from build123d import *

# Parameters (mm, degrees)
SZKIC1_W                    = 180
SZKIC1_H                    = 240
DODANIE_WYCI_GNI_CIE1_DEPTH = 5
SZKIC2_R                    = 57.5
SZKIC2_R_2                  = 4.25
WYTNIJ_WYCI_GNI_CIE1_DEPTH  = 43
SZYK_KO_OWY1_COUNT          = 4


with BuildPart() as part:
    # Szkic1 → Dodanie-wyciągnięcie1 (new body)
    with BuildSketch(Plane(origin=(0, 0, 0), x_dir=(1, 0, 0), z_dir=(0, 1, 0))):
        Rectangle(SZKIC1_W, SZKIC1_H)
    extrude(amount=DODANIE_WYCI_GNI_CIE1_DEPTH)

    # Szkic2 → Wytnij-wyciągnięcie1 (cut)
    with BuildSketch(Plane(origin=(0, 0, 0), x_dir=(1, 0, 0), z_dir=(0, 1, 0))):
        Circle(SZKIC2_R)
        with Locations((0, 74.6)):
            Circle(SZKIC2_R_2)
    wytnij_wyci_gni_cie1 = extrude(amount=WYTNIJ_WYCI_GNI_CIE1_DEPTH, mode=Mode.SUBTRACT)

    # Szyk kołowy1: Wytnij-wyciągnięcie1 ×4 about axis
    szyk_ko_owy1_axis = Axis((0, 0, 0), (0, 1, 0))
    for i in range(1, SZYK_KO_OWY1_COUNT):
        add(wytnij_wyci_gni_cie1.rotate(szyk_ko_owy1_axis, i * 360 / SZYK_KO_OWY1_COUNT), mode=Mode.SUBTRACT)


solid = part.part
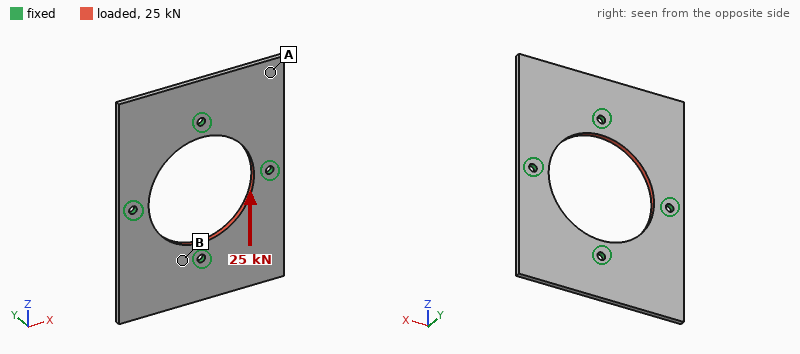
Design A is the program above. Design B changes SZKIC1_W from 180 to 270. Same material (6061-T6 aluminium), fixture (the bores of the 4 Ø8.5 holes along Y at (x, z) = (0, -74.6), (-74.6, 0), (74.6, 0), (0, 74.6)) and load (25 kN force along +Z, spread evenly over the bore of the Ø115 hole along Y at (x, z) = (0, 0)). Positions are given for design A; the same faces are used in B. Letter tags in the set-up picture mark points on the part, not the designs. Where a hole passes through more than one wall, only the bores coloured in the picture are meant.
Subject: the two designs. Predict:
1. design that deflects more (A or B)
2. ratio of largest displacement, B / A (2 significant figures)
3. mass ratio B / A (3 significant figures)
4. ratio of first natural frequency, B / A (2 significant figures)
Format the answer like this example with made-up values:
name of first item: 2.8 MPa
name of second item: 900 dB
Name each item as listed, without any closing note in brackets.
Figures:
design that deflects more: A
ratio of largest displacement, B / A: 0.88
mass ratio B / A: 1.66
ratio of first natural frequency, B / A: 0.59
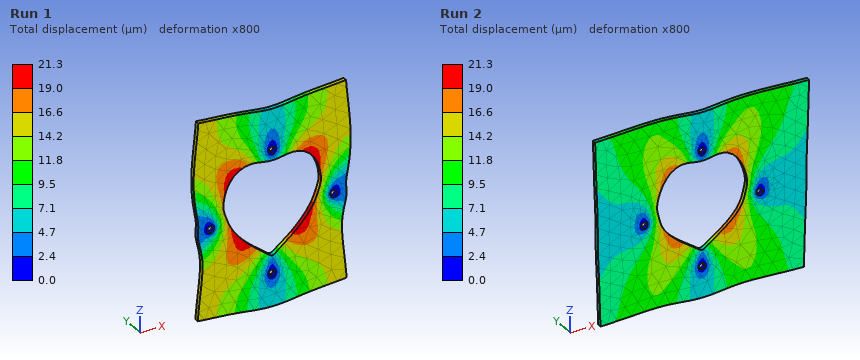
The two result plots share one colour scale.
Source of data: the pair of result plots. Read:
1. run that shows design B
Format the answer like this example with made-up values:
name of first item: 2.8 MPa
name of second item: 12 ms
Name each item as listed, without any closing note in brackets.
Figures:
run that shows design B: Run 2
